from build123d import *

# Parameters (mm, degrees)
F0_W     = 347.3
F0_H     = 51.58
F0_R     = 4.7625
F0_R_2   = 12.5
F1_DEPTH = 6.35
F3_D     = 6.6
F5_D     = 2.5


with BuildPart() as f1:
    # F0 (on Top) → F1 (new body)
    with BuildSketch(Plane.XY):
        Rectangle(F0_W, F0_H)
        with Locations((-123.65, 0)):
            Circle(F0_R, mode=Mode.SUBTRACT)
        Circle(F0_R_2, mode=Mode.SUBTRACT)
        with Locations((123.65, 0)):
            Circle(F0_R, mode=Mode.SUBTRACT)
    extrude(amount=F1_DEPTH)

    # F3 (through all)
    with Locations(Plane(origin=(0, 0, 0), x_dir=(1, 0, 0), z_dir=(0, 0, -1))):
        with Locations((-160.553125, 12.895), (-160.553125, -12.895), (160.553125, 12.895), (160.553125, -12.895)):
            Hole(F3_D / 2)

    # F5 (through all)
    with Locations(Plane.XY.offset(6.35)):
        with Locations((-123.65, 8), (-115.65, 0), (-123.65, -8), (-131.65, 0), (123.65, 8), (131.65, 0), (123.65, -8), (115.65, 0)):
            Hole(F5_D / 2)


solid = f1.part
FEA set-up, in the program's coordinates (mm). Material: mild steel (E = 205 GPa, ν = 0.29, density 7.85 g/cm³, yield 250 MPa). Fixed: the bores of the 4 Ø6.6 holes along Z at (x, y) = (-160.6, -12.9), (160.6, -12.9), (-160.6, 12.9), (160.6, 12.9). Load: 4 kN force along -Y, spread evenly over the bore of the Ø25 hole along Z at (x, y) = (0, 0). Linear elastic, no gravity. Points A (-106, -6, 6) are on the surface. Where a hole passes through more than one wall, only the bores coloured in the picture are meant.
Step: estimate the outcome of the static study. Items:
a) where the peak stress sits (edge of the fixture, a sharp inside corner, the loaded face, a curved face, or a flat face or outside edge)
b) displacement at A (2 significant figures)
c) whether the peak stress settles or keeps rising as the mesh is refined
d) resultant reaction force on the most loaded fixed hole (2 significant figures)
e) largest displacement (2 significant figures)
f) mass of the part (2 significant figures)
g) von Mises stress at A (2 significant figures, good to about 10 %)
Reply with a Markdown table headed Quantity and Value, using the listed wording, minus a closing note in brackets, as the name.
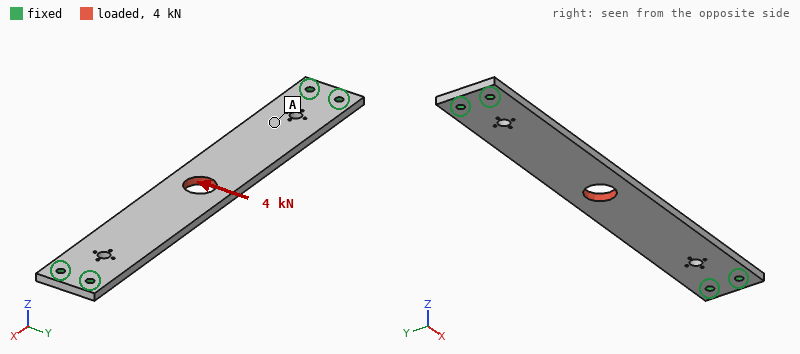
| Quantity | Value |
|---|---|
| where the peak stress sits | edge of the fixture |
| displacement at A | 22 µm |
| whether the peak stress settles or keeps rising as the mesh is refined | keeps rising |
| resultant reaction force on the most loaded fixed hole | 5.2 kN |
| largest displacement | 68 µm |
| mass of the part | 850 g |
| von Mises stress at A | 17 MPa |
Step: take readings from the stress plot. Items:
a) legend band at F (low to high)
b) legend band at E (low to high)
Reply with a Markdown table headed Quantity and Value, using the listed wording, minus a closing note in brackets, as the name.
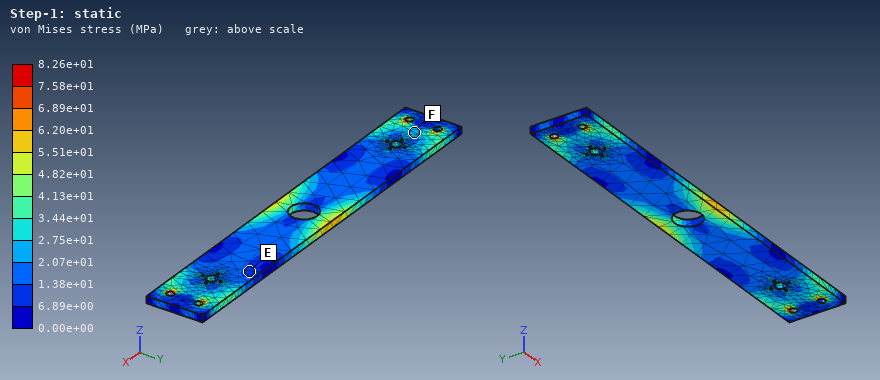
| Quantity | Value |
|---|---|
| legend band at F | 2.07e+01 to 2.75e+01 MPa |
| legend band at E | 6.89e+00 to 1.38e+01 MPa |
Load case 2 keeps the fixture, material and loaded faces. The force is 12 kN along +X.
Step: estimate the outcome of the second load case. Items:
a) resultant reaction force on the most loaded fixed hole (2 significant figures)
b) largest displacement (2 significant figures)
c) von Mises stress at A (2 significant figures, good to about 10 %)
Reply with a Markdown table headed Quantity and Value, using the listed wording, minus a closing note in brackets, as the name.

| Quantity | Value |
|---|---|
| resultant reaction force on the most loaded fixed hole | 3.0 kN |
| largest displacement | 15 µm |
| von Mises stress at A | 17 MPa |
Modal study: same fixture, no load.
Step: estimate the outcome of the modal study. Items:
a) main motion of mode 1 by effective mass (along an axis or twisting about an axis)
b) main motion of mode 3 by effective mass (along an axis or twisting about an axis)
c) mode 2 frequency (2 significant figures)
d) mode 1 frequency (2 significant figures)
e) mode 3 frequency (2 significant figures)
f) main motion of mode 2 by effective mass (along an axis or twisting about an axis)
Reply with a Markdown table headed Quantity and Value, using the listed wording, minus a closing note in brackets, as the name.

| Quantity | Value |
|---|---|
| main motion of mode 1 by effective mass | along Z |
| main motion of mode 3 by effective mass | twisting about X |
| mode 2 frequency | 900 Hz |
| mode 1 frequency | 320 Hz |
| mode 3 frequency | 1200 Hz |
| main motion of mode 2 by effective mass | twisting about Y |
